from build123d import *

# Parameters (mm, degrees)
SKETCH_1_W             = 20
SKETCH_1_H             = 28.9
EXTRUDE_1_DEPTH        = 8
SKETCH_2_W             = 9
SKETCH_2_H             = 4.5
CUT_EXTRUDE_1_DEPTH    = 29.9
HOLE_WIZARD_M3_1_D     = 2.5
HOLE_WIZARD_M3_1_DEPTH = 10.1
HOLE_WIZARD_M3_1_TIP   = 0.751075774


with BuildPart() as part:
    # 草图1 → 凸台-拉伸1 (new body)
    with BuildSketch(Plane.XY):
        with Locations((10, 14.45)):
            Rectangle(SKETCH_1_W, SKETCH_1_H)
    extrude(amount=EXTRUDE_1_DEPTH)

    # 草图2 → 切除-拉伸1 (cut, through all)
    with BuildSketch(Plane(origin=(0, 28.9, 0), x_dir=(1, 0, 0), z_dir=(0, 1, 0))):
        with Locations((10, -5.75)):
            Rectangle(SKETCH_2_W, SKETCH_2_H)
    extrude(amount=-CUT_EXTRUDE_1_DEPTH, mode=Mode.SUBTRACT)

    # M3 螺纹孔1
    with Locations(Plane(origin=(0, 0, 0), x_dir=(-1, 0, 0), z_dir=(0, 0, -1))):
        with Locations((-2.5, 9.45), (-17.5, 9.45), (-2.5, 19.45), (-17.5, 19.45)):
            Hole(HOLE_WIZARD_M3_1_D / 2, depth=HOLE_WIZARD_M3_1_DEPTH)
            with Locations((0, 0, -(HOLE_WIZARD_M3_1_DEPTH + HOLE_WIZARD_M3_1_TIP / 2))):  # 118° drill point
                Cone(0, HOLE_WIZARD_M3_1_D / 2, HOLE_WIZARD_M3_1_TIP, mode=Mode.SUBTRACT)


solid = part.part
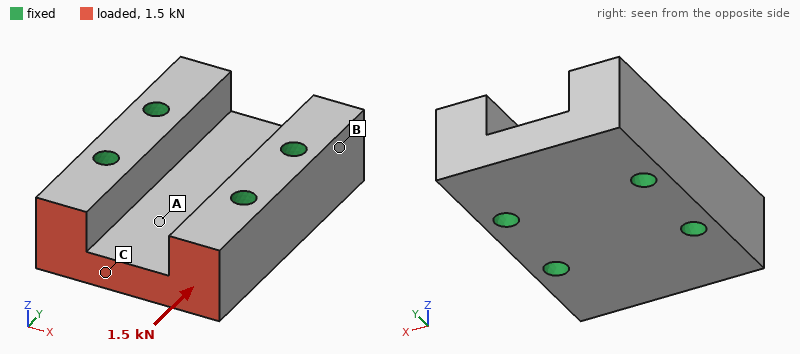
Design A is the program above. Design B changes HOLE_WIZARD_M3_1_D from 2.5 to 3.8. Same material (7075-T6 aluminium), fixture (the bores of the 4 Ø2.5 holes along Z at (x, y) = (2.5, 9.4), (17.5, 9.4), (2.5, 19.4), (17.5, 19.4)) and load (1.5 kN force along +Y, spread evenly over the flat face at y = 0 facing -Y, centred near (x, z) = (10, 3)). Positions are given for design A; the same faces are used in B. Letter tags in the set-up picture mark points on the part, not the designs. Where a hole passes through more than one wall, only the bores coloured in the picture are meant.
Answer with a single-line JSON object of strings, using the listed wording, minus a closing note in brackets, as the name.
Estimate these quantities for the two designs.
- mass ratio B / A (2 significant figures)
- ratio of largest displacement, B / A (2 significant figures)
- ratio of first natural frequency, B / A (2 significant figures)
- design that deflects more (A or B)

{"mass ratio B / A": "0.94", "ratio of largest displacement, B / A": "0.90", "ratio of first natural frequency, B / A": "1.1", "design that deflects more": "A"}
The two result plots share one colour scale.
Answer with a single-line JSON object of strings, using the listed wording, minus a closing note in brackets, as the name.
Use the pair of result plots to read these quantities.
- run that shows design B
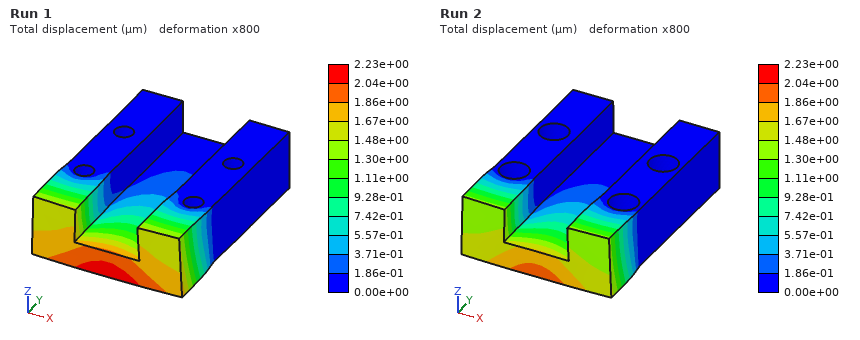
{"run that shows design B": "Run 2"}
